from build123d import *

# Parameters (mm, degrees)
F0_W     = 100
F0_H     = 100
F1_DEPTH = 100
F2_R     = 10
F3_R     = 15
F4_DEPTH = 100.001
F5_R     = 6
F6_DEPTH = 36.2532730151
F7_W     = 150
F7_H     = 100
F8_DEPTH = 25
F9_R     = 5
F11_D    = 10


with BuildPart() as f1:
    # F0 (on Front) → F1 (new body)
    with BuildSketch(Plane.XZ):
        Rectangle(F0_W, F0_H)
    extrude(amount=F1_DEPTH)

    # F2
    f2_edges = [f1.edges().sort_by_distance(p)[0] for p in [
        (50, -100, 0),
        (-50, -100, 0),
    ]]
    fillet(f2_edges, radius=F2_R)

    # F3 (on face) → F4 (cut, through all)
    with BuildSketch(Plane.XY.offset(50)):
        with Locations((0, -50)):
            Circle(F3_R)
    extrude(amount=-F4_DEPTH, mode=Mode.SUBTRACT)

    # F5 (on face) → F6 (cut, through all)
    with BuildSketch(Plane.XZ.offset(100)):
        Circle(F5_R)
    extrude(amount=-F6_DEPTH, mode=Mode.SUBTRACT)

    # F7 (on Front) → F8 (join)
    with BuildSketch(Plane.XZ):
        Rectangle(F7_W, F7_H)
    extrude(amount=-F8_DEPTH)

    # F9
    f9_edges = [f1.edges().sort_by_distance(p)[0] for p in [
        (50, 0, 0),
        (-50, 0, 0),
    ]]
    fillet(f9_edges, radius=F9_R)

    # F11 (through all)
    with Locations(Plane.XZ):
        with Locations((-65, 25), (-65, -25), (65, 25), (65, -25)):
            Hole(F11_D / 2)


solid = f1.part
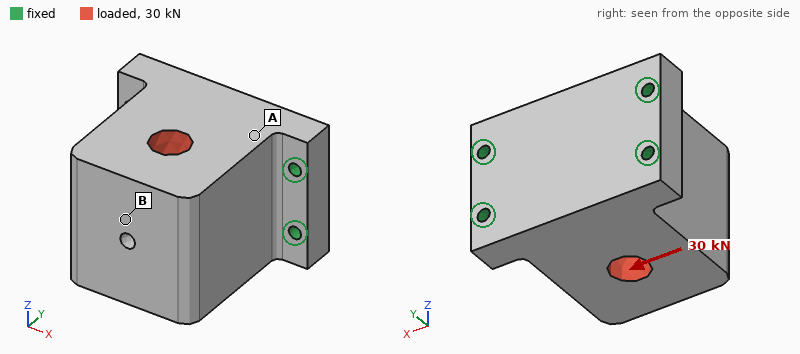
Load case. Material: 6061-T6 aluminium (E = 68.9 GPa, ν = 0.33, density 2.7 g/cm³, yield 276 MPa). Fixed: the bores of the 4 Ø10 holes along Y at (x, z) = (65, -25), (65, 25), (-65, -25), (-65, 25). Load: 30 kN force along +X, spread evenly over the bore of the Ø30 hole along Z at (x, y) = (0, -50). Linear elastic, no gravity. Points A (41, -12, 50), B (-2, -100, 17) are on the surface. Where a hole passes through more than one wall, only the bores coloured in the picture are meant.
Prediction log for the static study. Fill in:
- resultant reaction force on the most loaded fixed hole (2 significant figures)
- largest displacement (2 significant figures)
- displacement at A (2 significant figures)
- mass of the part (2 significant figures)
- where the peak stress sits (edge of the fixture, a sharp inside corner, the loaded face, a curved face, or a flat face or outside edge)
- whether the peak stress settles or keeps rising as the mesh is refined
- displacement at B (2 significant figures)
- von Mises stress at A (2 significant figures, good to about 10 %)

11 kN
35 µm
10.0 µm
3.5 kg
edge of the fixture
keeps rising
33 µm
7.6 MPa
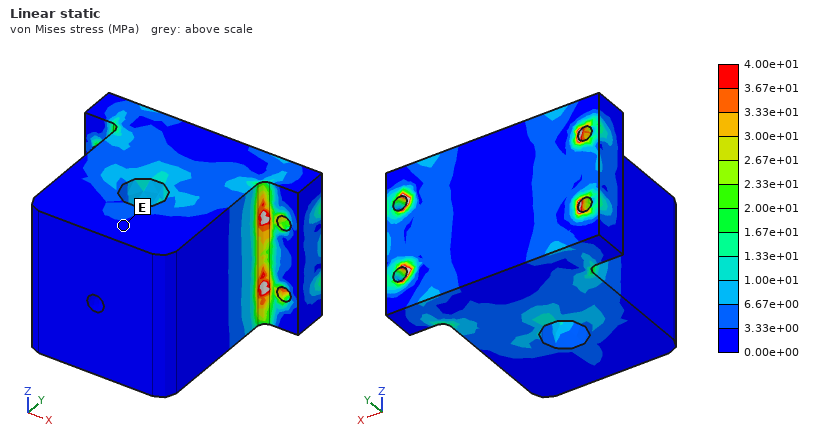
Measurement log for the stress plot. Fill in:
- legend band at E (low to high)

0.00e+00 to 3.33e+00 MPa
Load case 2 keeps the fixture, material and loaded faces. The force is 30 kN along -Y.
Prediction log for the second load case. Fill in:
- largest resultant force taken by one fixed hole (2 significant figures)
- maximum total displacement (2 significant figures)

8.2 kN
15 µm
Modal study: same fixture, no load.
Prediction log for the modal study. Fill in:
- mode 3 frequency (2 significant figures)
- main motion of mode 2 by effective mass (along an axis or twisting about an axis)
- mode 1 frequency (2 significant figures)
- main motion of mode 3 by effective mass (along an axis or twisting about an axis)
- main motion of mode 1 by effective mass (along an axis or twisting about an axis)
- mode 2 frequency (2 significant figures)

4400 Hz
along X
1900 Hz
along Y
along Z
3300 Hz
